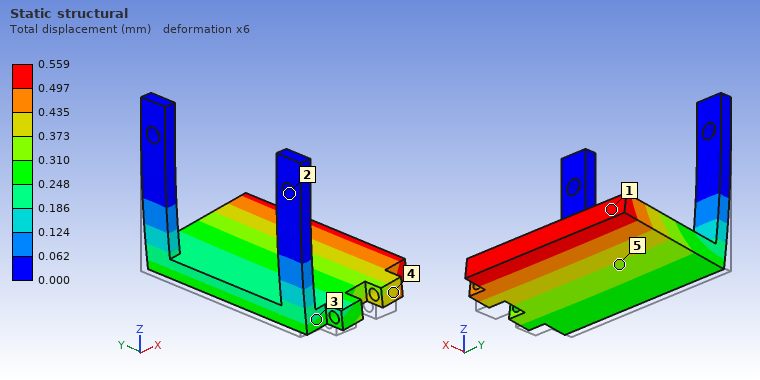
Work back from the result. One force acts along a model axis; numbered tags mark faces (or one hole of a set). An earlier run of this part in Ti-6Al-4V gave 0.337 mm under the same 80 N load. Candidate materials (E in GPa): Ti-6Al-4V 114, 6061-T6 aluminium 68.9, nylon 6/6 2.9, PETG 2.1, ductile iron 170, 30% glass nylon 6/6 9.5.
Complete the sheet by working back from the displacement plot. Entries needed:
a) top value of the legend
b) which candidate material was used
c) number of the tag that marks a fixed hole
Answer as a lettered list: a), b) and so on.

a) 0.559 mm
b) 6061-T6 aluminium
c) 2
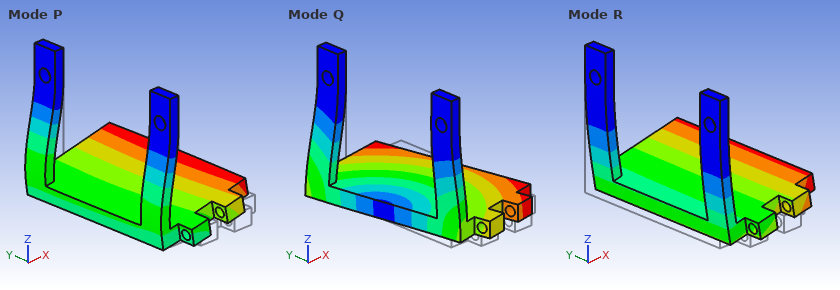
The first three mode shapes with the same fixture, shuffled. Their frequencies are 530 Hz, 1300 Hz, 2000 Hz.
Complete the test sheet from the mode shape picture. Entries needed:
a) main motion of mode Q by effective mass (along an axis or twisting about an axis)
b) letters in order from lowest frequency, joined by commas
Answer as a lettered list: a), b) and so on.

a) along Y
b) R, Q, P
